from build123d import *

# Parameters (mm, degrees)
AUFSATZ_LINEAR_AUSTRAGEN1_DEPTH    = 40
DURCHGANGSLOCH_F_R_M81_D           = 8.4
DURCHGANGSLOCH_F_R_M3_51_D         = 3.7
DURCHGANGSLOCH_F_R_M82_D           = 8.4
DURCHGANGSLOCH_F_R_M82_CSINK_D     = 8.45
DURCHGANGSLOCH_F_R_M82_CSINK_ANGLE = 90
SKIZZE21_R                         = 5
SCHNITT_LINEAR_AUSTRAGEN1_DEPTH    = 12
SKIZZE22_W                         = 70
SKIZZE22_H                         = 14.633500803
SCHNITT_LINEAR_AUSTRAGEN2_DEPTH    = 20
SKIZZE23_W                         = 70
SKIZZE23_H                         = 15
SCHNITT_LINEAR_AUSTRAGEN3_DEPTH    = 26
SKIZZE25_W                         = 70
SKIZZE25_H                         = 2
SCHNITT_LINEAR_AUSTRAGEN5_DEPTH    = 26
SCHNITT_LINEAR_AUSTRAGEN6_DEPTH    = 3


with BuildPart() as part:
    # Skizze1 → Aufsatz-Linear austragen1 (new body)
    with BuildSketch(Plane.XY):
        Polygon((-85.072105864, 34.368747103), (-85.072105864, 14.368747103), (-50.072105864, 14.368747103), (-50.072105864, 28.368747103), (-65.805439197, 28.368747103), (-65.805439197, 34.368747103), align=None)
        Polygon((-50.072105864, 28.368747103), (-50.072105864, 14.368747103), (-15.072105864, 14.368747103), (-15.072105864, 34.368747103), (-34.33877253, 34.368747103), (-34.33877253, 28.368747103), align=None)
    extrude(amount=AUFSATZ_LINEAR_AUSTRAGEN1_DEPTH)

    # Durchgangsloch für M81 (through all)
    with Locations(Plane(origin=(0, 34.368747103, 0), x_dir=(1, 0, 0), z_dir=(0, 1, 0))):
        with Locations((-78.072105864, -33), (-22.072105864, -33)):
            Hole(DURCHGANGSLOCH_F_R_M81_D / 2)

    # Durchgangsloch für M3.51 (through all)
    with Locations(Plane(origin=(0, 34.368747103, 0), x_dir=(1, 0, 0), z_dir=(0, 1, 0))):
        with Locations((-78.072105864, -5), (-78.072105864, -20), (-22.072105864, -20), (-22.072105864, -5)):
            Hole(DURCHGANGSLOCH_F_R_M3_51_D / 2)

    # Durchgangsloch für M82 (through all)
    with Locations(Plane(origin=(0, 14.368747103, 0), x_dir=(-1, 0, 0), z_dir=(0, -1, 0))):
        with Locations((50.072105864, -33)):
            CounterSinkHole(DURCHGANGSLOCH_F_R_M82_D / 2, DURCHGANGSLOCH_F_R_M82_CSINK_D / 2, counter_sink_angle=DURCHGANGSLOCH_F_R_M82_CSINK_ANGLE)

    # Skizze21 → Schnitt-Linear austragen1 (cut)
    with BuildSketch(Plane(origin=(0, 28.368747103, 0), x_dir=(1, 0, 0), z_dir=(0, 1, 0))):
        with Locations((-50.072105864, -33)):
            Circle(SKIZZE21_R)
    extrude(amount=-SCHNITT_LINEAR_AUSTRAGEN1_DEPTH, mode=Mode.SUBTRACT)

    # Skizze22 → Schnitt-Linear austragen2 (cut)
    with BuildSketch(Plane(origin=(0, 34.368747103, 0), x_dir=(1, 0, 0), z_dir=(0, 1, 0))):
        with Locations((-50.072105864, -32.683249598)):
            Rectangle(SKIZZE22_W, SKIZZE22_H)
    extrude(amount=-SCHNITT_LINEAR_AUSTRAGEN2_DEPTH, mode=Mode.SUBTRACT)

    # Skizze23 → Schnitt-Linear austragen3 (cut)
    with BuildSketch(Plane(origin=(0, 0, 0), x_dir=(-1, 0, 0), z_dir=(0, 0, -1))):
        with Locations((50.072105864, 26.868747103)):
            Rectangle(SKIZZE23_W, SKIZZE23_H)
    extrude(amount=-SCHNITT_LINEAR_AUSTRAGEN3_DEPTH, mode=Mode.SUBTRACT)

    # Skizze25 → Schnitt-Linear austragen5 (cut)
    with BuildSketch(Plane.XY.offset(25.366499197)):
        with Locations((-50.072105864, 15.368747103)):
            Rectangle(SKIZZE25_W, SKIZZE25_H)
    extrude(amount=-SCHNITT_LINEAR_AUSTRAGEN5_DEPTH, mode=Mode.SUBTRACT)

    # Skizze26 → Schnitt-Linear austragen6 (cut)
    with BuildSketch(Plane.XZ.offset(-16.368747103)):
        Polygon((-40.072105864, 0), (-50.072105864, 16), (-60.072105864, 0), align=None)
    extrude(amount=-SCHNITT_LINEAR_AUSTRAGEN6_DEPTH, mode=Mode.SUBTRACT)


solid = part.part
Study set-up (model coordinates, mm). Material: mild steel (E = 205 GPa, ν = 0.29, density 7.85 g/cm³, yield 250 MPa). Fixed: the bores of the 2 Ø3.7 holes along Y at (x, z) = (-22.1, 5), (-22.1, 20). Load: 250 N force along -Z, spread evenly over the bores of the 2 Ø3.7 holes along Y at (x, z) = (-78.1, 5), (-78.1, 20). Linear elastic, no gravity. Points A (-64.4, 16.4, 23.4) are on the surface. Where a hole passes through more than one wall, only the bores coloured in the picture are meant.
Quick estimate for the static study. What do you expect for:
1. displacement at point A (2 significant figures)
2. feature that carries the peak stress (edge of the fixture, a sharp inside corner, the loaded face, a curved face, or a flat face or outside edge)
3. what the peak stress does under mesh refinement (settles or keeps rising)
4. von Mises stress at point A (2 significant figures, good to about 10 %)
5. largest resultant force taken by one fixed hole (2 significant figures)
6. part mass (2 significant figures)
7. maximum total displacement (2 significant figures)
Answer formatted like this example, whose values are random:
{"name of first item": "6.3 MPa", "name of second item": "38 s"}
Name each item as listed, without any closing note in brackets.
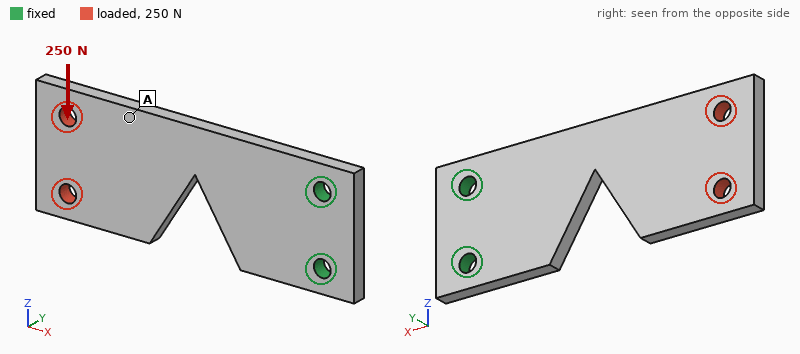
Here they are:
{"displacement at point A": "41 µm", "feature that carries the peak stress": "a sharp inside corner", "what the peak stress does under mesh refinement": "keeps rising", "von Mises stress at point A": "19 MPa", "largest resultant force taken by one fixed hole": "840 N", "part mass": "37 g", "maximum total displacement": "96 µm"}
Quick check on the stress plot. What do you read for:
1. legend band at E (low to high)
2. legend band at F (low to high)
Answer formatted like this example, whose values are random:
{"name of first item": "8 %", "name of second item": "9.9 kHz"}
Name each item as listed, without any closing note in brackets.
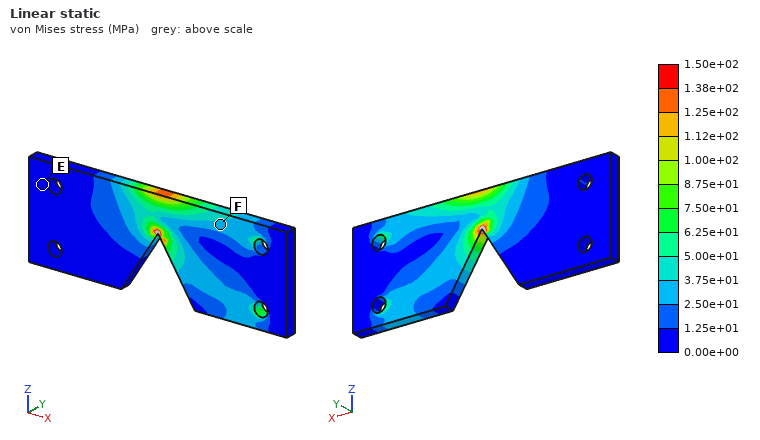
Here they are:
{"legend band at E": "0.00e+00 to 1.25e+01 MPa", "legend band at F": "2.50e+01 to 3.75e+01 MPa"}
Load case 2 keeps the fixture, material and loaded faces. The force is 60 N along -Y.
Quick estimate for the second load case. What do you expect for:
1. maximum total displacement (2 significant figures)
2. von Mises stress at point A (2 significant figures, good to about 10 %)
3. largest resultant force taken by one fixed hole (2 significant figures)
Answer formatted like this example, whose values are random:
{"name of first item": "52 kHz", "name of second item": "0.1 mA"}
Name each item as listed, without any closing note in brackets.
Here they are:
{"maximum total displacement": "0.48 mm", "von Mises stress at point A": "32 MPa", "largest resultant force taken by one fixed hole": "31 N"}
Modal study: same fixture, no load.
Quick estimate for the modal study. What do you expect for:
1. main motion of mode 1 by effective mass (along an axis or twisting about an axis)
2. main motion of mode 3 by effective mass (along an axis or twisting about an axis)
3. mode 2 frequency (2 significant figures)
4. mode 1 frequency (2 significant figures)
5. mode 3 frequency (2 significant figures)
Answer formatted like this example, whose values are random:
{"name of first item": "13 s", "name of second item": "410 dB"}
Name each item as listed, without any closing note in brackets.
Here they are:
{"main motion of mode 1 by effective mass": "along Y", "main motion of mode 3 by effective mass": "along Z", "mode 2 frequency": "2600 Hz", "mode 1 frequency": "580 Hz", "mode 3 frequency": "2700 Hz"}
